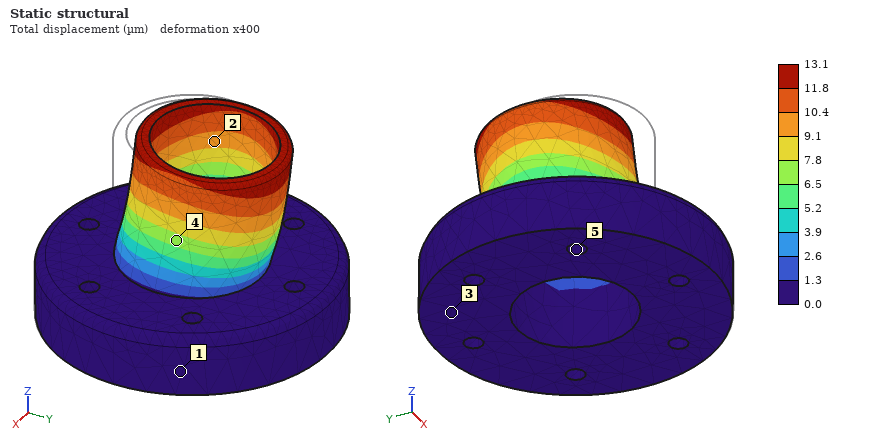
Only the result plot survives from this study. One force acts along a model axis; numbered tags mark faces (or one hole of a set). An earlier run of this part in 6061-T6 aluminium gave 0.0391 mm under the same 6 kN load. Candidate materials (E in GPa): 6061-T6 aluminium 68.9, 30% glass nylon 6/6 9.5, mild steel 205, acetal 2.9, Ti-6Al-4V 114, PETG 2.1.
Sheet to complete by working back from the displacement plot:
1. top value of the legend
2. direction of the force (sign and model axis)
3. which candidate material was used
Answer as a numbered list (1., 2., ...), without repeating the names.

1. 13.1 µm
2. +Y
3. mild steel
